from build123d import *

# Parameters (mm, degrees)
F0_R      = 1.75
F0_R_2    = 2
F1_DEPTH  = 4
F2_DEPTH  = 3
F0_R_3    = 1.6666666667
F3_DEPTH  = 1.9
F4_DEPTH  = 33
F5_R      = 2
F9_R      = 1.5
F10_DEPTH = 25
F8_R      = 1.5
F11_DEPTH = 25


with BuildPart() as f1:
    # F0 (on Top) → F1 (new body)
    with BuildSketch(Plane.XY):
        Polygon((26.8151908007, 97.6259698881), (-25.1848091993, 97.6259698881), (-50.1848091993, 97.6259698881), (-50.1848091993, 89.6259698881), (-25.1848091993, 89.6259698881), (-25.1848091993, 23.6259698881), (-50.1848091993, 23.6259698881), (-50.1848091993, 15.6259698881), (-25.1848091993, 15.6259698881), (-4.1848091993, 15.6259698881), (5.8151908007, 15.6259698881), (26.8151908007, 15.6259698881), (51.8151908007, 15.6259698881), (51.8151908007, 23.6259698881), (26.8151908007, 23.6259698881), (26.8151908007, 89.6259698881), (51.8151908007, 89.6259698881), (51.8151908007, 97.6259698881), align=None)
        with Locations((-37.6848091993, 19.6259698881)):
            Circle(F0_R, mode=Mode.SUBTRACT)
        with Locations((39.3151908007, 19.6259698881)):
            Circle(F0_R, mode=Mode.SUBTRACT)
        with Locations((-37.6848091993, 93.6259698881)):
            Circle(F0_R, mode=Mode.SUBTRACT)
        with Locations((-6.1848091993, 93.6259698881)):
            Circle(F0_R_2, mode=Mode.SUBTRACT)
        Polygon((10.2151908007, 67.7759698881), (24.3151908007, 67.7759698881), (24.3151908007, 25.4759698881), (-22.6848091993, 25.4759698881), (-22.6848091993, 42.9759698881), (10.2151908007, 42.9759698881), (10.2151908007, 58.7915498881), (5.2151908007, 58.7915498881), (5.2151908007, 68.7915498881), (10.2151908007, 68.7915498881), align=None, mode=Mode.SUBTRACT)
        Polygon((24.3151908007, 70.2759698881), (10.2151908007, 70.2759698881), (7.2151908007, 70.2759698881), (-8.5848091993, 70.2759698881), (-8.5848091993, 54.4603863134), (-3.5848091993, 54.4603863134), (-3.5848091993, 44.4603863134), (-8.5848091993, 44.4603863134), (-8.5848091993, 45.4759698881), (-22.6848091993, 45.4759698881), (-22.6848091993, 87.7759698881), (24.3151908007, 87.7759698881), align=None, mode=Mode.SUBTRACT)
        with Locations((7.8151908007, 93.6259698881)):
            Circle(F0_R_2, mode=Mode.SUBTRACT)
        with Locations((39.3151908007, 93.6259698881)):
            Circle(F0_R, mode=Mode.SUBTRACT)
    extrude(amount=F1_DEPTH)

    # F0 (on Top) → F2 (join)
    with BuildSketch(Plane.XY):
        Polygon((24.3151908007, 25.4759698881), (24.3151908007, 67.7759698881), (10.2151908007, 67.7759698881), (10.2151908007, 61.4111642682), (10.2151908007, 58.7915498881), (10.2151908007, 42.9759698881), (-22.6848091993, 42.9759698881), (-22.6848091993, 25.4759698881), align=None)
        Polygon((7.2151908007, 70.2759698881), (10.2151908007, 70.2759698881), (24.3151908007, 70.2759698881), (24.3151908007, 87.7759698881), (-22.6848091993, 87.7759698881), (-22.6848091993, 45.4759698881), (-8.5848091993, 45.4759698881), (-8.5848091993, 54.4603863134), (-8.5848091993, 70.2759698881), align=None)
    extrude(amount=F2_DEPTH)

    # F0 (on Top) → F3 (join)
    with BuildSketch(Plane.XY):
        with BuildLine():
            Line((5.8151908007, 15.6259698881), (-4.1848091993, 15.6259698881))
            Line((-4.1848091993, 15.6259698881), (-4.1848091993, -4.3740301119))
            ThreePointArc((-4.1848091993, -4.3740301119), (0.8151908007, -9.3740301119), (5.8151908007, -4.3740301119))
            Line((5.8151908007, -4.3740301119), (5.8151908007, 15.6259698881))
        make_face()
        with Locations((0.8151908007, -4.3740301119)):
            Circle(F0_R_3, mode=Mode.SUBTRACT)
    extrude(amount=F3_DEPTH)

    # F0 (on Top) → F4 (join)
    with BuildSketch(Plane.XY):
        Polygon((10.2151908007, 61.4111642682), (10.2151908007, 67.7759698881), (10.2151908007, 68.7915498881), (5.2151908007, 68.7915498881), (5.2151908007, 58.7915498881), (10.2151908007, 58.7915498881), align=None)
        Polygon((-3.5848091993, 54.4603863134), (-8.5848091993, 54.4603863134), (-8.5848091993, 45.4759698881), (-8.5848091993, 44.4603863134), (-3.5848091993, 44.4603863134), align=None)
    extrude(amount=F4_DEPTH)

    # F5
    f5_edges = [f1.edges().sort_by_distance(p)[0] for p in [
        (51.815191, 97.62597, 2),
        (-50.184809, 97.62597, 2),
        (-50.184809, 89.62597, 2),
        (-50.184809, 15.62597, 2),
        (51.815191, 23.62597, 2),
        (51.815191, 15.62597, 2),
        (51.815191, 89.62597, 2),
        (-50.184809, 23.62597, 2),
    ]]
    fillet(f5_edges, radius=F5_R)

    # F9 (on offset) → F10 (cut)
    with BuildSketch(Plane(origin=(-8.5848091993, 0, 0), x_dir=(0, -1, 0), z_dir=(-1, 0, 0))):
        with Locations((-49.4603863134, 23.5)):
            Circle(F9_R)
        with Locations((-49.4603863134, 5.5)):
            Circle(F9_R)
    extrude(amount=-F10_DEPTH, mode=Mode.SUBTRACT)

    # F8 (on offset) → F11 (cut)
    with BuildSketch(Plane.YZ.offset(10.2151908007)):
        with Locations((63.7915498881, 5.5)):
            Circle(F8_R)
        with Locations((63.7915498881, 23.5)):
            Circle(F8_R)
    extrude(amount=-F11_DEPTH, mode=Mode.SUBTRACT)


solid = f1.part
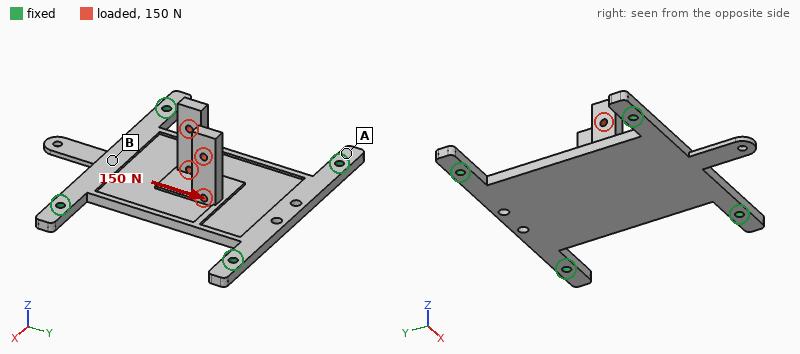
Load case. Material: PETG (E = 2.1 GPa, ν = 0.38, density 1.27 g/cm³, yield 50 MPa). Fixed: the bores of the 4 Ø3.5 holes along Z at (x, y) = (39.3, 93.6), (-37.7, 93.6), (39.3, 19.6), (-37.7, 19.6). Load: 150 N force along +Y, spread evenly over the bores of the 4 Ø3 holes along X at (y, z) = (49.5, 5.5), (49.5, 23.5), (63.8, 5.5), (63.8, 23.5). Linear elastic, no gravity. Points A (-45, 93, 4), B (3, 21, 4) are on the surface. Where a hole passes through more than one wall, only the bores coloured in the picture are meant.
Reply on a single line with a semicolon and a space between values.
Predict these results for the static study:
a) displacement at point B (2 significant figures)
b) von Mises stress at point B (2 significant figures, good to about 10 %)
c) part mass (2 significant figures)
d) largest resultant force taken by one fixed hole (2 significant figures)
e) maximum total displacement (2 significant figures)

0.34 mm; 3.2 MPa; 26 g; 45 N; 1.3 mm
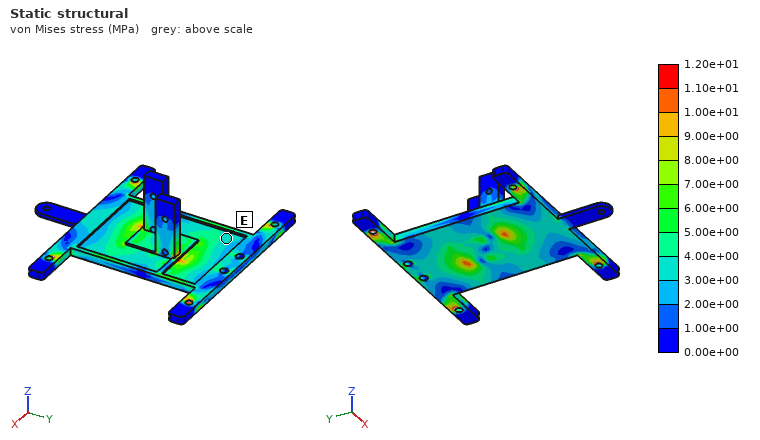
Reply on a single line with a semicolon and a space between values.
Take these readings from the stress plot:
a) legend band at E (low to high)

3.00e+00 to 4.00e+00 MPa
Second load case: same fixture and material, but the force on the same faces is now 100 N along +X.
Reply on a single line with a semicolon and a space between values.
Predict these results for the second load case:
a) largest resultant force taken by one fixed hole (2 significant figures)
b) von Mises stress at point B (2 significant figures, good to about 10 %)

28 N; 3.1 MPa
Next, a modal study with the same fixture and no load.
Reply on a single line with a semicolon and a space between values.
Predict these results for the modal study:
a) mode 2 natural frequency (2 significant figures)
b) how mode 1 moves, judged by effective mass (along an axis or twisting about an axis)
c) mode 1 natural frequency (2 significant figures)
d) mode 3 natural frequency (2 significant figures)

530 Hz; along Z; 370 Hz; 580 Hz
